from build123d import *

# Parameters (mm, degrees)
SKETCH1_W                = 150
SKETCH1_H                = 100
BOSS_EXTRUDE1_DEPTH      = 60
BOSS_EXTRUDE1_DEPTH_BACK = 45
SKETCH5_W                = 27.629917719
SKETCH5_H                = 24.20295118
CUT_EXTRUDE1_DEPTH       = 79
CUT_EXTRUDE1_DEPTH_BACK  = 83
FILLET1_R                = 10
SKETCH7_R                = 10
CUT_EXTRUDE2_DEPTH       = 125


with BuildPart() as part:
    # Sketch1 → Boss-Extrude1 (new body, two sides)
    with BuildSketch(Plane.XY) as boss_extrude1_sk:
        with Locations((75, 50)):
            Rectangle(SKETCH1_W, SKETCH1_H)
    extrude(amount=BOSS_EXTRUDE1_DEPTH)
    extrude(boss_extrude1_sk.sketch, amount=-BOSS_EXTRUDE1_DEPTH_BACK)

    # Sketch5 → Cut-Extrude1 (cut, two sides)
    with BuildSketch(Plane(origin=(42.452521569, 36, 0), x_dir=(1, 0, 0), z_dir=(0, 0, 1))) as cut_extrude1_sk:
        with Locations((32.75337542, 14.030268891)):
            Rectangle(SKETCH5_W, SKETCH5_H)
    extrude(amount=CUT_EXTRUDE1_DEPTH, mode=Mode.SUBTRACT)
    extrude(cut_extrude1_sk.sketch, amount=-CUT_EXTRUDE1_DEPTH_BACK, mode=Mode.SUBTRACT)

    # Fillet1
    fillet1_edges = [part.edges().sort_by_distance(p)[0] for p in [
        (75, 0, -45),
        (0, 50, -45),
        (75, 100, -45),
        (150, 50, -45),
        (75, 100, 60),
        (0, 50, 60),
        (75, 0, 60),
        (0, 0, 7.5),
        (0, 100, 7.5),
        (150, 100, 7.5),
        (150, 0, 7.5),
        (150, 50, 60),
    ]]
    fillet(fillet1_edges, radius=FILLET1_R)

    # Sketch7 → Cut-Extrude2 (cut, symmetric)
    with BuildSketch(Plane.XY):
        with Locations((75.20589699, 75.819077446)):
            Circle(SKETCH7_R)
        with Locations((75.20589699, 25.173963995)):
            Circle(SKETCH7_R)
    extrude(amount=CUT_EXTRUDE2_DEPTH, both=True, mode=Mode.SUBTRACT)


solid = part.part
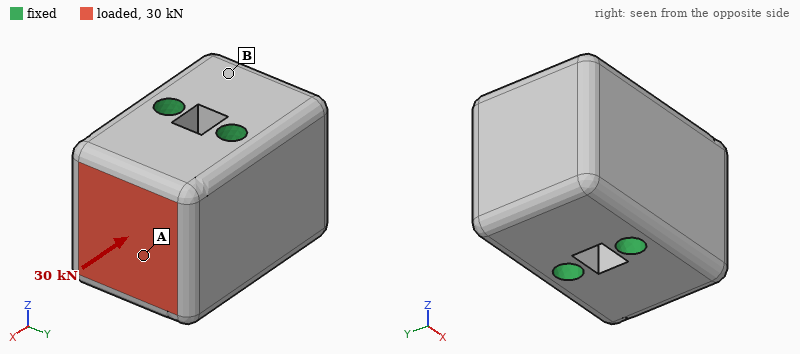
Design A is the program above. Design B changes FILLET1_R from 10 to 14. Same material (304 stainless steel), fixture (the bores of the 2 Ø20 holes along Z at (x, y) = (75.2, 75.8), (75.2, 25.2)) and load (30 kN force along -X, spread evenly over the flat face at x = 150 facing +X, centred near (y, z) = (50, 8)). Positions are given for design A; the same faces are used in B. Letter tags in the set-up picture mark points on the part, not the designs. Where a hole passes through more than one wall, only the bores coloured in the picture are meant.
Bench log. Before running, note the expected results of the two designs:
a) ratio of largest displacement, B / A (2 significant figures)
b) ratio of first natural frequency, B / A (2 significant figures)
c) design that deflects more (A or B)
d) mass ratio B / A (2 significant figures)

1.1
1.0
B
0.98
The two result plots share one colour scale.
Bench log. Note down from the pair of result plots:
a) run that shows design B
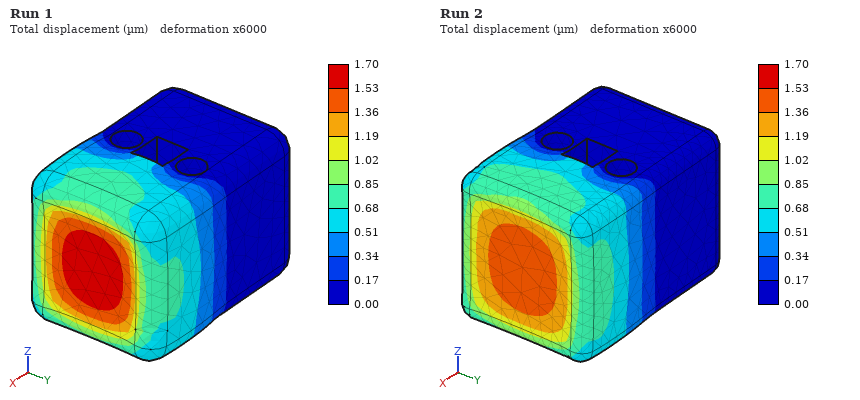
Run 1
